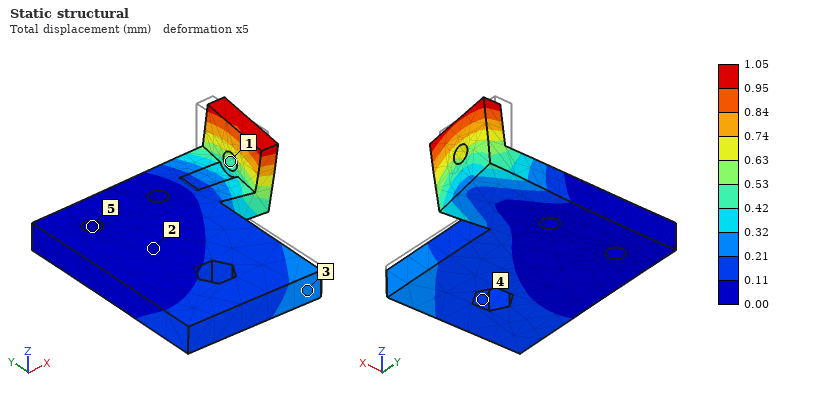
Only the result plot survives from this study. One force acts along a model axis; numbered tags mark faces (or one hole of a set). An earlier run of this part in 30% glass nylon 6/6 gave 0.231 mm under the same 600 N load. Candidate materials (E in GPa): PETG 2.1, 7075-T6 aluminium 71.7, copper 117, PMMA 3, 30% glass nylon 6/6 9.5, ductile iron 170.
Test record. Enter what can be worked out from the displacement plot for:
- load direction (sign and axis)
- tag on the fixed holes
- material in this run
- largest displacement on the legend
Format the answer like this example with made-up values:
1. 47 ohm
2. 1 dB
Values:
1. -Y
2. 5
3. PETG
4. 1.05 mm
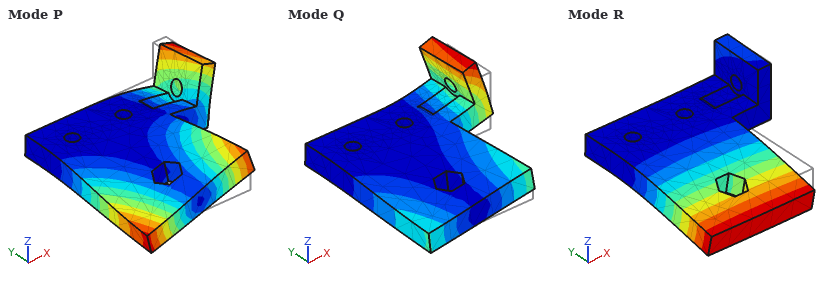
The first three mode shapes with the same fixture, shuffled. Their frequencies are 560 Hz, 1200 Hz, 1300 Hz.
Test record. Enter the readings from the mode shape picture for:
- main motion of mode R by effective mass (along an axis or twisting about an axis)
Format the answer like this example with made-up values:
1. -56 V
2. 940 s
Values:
1. along Z
